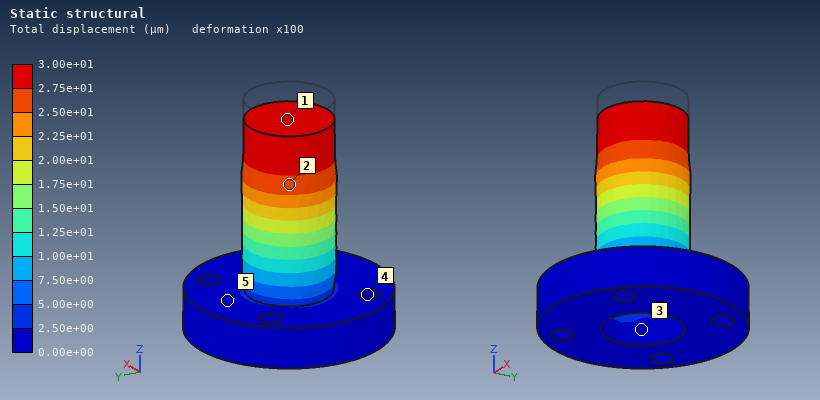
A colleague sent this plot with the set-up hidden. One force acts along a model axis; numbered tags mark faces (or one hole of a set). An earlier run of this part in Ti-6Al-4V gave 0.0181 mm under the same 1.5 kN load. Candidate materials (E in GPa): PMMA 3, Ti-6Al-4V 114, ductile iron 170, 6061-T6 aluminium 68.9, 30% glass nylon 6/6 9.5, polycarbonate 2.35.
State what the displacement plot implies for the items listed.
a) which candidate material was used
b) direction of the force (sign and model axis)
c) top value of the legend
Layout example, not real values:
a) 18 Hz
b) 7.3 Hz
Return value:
a) 6061-T6 aluminium
b) -Z
c) 3.00e+01 µm
